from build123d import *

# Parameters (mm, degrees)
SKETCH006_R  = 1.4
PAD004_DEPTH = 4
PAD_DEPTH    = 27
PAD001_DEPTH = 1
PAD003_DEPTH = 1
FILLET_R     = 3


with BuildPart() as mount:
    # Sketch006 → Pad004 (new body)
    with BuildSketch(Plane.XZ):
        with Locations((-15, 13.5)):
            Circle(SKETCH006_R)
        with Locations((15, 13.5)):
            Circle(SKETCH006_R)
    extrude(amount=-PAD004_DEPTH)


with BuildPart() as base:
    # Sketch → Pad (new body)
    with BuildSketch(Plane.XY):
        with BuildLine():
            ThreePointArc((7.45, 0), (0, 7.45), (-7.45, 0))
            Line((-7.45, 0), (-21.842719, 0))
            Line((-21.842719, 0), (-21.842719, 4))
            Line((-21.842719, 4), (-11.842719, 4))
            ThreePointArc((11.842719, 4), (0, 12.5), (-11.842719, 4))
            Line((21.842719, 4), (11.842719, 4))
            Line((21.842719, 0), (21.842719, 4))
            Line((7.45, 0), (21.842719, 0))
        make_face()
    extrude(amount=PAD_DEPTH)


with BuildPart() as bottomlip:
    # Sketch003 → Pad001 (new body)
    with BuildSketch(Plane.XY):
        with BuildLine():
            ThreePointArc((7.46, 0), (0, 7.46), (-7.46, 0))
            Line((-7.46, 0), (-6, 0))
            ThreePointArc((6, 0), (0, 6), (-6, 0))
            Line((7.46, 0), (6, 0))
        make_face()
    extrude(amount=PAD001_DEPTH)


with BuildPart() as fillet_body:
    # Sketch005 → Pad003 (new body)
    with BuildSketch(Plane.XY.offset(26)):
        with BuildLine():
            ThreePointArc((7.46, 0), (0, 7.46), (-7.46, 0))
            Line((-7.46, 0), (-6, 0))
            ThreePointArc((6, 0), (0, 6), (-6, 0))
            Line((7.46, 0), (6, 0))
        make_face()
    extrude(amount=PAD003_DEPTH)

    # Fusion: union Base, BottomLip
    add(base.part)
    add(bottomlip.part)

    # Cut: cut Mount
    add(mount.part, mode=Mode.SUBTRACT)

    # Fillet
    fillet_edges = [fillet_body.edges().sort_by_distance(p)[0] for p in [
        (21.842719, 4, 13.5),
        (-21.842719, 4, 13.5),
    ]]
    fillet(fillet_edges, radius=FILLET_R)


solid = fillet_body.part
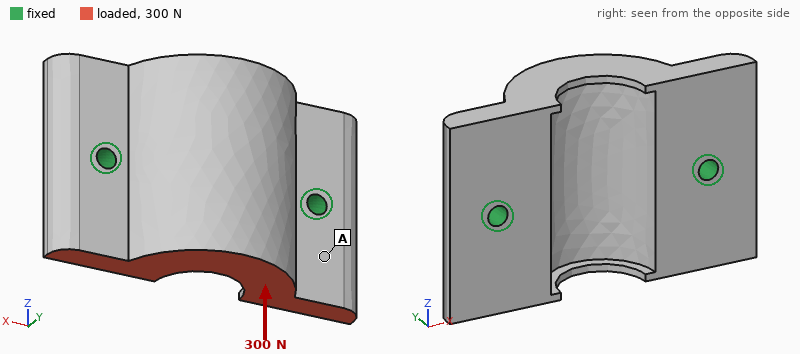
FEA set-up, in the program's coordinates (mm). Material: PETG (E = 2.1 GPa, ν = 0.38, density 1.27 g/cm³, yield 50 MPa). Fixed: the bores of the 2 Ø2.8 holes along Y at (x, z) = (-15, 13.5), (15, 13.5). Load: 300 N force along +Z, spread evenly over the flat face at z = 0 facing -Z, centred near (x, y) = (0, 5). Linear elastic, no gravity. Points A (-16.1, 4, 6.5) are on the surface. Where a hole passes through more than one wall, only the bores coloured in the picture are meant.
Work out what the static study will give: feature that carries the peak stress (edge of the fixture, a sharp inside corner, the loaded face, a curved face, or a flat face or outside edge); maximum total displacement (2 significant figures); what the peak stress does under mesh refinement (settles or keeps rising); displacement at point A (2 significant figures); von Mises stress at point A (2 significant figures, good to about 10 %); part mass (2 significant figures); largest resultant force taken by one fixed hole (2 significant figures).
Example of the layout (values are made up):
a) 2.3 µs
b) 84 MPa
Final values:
a) edge of the fixture
b) 0.20 mm
c) keeps rising
d) 0.042 mm
e) 3.9 MPa
f) 7.9 g
g) 150 N
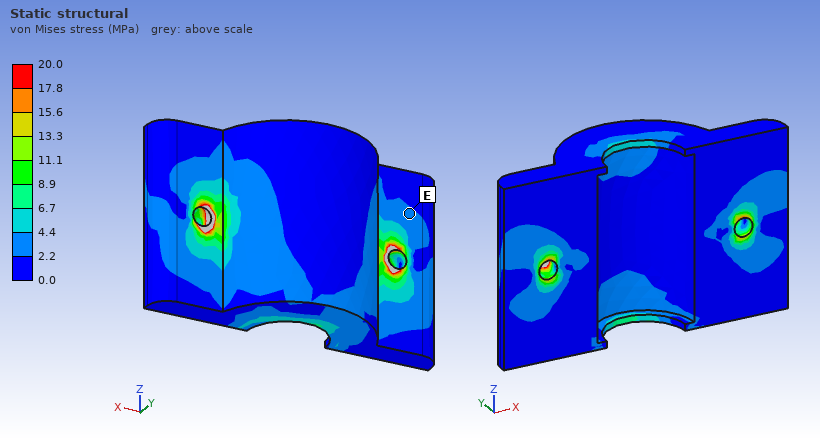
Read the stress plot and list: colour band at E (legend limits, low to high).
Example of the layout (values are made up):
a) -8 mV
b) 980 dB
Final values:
a) 2.2 to 4.4 MPa
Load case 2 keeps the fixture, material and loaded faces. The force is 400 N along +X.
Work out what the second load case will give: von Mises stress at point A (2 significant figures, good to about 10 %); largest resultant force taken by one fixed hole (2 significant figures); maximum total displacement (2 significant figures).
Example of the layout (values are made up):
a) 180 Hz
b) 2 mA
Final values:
a) 6.0 MPa
b) 260 N
c) 0.19 mm
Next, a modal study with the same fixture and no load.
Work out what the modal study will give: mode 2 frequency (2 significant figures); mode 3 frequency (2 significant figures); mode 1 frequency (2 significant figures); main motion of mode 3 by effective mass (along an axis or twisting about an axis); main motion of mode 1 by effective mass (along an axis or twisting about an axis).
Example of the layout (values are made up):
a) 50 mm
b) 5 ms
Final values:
a) 4600 Hz
b) 5000 Hz
c) 2100 Hz
d) along Y
e) along Z
